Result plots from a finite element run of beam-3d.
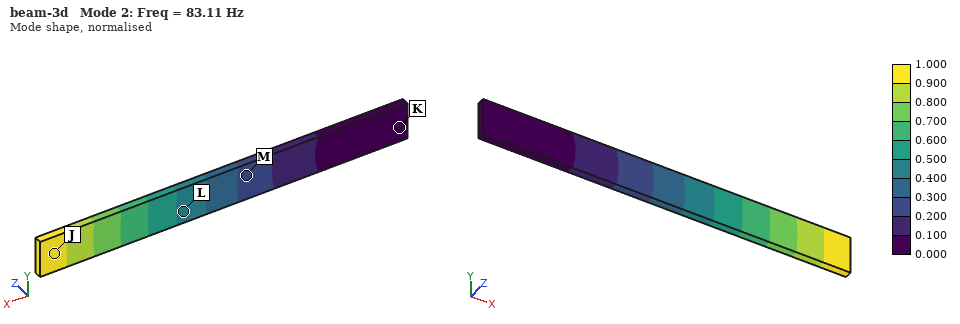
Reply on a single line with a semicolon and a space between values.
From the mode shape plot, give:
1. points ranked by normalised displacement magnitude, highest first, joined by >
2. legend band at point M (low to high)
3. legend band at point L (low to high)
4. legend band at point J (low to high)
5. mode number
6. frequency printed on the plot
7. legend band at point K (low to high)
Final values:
J > L > M > K; 0.200 to 0.300; 0.400 to 0.500; 0.900 to 1.000; 2; 83.11 Hz; 0.000 to 0.100
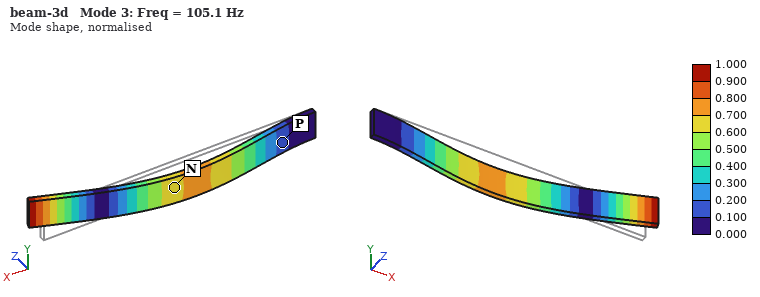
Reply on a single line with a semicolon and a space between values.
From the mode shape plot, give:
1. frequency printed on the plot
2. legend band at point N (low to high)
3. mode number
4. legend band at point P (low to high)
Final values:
105.1 Hz; 0.600 to 0.700; 3; 0.100 to 0.200
